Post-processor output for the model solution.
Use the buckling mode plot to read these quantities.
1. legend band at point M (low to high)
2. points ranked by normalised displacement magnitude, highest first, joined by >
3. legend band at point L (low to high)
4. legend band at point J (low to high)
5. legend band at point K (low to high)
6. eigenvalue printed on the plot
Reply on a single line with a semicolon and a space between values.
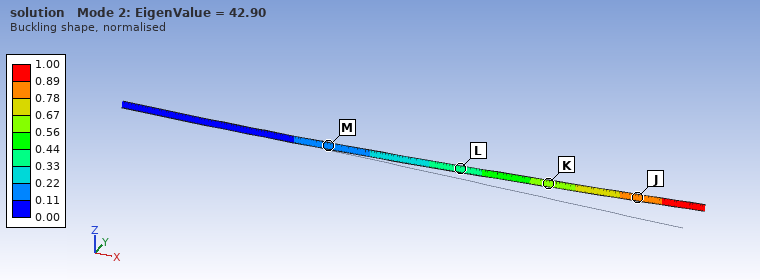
0.11 to 0.22; J > K > L > M; 0.33 to 0.44; 0.78 to 0.89; 0.56 to 0.67; 42.90
